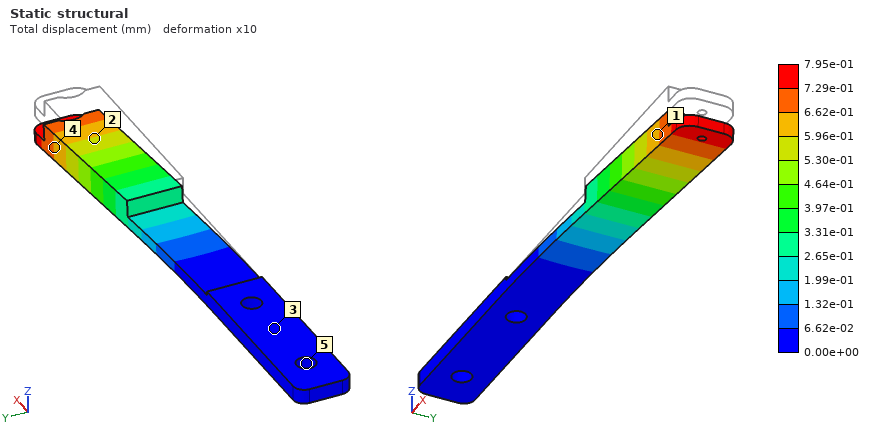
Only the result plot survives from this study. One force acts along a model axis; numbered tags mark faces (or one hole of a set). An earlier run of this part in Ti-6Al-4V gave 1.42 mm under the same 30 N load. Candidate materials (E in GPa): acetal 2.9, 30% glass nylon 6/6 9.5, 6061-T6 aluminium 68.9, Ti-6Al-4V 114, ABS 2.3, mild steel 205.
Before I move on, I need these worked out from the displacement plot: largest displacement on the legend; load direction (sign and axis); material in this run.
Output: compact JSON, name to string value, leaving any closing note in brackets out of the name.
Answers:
{"largest displacement on the legend": "7.95e-01 mm", "load direction": "-Z", "material in this run": "mild steel"}
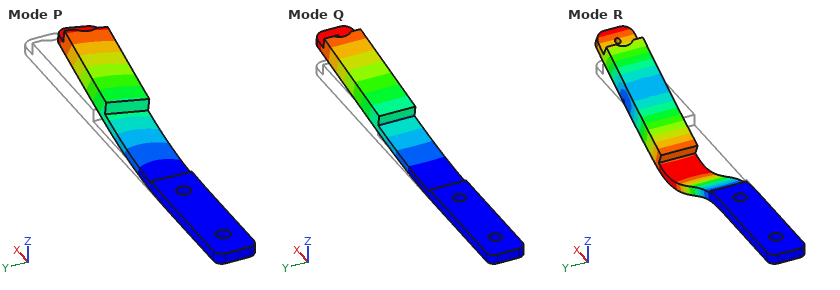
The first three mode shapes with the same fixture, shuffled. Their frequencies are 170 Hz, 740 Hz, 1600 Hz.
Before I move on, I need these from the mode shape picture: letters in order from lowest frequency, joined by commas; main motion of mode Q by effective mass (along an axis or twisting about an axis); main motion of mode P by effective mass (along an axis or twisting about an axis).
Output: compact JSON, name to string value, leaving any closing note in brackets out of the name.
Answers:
{"letters in order from lowest frequency, joined by commas": "Q, P, R", "main motion of mode Q by effective mass": "along Z", "main motion of mode P by effective mass": "along Y"}
